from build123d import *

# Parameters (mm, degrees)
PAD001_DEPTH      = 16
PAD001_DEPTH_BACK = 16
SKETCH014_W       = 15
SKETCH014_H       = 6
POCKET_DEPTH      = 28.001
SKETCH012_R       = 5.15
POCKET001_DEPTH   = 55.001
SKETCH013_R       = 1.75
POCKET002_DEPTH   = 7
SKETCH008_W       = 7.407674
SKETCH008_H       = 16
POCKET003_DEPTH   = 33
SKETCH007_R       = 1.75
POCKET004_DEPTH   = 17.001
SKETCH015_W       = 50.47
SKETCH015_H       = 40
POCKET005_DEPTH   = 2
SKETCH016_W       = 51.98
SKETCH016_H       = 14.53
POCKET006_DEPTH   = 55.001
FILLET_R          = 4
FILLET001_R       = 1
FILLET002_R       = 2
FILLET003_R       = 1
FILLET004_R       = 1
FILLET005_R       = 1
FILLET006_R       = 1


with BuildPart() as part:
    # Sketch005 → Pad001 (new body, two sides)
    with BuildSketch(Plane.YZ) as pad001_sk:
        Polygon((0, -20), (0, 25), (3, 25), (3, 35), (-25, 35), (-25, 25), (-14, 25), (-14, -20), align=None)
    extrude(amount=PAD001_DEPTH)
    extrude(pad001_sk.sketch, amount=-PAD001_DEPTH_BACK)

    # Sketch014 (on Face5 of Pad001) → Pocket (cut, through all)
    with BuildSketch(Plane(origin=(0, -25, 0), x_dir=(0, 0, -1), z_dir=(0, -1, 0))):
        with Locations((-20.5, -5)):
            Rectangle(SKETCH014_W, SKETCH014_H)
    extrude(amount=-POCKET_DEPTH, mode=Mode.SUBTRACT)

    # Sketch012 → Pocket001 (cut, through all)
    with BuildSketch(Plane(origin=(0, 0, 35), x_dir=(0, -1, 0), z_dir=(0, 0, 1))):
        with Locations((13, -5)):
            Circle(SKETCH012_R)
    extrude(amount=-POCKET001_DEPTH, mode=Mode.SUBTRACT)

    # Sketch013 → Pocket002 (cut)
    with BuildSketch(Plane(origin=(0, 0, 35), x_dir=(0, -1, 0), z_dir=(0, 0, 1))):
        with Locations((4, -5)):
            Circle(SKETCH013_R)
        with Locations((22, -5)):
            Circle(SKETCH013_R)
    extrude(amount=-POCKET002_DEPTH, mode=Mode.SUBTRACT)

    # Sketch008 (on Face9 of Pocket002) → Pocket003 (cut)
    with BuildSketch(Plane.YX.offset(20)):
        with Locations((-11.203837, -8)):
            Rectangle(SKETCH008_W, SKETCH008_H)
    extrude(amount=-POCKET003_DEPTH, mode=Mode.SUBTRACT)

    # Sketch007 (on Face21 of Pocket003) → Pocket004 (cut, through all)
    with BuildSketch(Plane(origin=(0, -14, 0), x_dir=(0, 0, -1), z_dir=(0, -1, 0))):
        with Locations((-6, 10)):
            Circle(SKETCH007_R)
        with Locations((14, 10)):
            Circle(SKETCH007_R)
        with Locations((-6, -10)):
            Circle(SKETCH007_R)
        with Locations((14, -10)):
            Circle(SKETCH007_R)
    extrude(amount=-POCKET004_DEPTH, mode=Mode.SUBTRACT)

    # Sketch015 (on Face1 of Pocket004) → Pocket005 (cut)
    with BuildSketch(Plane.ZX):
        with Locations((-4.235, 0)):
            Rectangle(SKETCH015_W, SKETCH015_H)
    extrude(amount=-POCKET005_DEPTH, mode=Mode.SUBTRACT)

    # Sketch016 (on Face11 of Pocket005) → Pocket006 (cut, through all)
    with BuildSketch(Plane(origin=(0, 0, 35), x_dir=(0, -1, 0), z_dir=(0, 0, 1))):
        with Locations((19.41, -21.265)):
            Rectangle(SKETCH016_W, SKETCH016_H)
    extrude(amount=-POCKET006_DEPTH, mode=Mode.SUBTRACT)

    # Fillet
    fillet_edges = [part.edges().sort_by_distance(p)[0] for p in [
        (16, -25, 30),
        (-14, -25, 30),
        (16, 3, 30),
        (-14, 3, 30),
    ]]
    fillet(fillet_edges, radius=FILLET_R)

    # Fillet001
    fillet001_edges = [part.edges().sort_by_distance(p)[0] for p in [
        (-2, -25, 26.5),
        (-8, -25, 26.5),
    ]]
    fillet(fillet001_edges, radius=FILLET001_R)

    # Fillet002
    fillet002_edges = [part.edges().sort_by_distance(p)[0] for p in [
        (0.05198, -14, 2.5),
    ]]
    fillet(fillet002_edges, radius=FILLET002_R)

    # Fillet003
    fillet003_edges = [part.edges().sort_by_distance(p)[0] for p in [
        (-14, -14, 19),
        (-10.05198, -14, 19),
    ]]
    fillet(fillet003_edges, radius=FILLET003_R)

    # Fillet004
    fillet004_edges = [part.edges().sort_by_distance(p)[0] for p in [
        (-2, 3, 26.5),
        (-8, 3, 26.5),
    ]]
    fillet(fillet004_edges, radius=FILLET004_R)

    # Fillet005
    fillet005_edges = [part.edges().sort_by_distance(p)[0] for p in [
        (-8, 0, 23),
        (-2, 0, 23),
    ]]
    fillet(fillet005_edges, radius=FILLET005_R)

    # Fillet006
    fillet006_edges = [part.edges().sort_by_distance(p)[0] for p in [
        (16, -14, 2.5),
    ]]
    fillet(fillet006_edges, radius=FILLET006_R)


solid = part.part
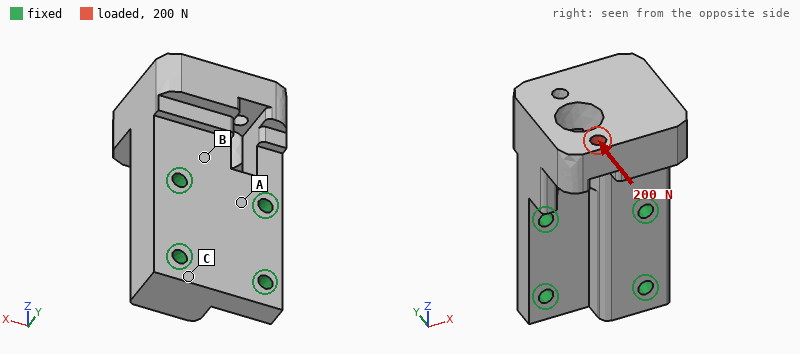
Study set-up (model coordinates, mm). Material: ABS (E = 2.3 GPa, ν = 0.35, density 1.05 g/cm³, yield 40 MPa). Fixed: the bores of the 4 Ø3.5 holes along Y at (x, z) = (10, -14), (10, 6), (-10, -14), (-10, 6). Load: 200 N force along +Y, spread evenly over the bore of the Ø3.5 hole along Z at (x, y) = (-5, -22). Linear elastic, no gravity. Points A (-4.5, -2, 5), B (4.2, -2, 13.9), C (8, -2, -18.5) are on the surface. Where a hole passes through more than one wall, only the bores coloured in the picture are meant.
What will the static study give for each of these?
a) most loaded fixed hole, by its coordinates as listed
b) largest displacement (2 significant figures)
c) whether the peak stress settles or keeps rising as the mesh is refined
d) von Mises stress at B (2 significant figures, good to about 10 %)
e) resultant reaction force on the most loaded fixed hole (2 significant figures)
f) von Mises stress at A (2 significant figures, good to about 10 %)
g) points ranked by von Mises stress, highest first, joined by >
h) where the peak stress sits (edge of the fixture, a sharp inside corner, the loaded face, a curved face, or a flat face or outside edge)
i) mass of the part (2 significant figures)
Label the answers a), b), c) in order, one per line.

a) (10, 6)
b) 0.52 mm
c) keeps rising
d) 8.3 MPa
e) 170 N
f) 3.9 MPa
g) B > A > C
h) edge of the fixture
i) 20 g
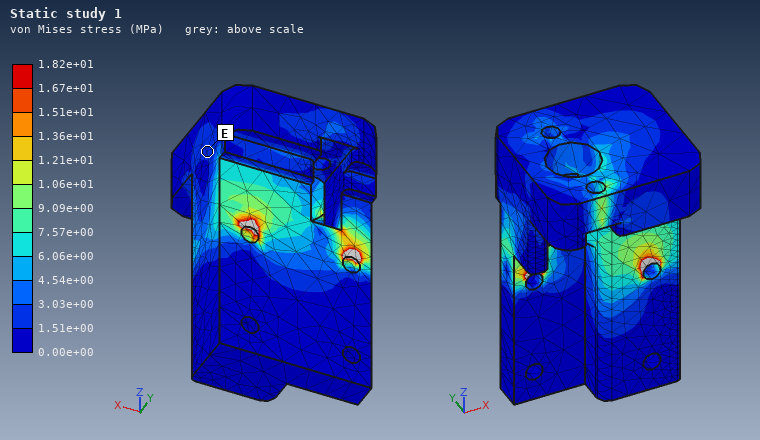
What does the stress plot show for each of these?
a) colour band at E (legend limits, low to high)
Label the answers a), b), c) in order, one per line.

a) 1.51e+00 to 3.03e+00 MPa
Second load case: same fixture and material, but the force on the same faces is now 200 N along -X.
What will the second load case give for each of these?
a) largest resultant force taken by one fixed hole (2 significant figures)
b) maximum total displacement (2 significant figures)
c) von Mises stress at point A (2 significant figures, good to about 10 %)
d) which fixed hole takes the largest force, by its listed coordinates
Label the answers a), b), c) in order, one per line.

a) 290 N
b) 0.28 mm
c) 2.1 MPa
d) (10, 6)
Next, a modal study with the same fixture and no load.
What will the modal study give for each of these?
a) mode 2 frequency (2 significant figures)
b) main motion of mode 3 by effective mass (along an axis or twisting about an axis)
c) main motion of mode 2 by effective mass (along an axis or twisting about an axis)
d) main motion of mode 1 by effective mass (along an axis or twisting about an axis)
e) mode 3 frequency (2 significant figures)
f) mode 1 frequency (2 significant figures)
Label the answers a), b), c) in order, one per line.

a) 2400 Hz
b) along X
c) along X
d) along Y
e) 3200 Hz
f) 1500 Hz
